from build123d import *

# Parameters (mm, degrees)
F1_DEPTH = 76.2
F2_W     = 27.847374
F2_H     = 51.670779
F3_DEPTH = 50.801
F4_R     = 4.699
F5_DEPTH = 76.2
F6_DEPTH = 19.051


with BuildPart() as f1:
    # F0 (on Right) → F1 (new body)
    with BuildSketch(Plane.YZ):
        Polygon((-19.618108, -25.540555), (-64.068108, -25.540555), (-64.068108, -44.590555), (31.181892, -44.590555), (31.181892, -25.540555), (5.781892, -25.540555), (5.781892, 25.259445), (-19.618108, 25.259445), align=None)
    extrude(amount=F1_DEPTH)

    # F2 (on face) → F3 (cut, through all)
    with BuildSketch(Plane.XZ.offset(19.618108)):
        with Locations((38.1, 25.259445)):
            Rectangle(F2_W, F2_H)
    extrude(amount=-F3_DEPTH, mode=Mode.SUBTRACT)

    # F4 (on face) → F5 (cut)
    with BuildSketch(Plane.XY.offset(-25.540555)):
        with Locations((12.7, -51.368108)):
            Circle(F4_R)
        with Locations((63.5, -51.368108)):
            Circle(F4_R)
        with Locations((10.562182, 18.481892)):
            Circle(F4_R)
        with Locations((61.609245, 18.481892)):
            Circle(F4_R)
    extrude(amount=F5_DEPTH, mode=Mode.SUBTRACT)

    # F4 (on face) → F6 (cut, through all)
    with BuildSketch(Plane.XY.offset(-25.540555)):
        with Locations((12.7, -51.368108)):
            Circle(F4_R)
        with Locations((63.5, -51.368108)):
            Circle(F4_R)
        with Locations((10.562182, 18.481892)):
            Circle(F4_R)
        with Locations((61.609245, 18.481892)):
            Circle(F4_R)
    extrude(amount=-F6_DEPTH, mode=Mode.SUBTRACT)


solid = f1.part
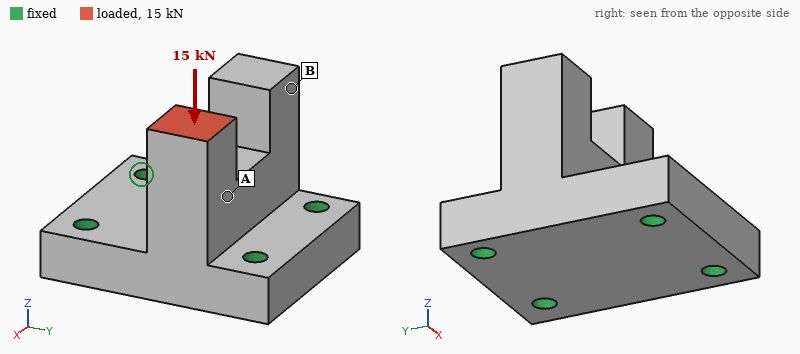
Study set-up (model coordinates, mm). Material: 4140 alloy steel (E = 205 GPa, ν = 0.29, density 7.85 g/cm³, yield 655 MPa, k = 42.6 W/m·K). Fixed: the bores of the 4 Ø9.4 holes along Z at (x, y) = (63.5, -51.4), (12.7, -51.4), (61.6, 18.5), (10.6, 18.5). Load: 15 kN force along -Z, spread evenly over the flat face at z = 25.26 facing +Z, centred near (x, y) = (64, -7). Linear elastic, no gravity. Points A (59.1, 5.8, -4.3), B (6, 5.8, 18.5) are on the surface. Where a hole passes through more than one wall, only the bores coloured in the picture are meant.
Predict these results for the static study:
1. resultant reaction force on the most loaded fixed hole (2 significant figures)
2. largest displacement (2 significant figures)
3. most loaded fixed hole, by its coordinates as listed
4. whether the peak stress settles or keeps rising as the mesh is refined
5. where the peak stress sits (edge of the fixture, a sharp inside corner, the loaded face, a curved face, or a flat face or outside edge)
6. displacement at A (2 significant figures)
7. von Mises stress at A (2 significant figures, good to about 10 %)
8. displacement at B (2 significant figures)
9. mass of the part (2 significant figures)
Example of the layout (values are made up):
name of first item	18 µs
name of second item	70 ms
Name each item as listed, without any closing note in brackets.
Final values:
resultant reaction force on the most loaded fixed hole	10 kN
largest displacement	20 µm
most loaded fixed hole, by its coordinates as listed	(61.6, 18.5)
whether the peak stress settles or keeps rising as the mesh is refined	keeps rising
where the peak stress sits	edge of the fixture
displacement at A	8.7 µm
von Mises stress at A	22 MPa
displacement at B	6.6 µm
mass of the part	1.7 kg
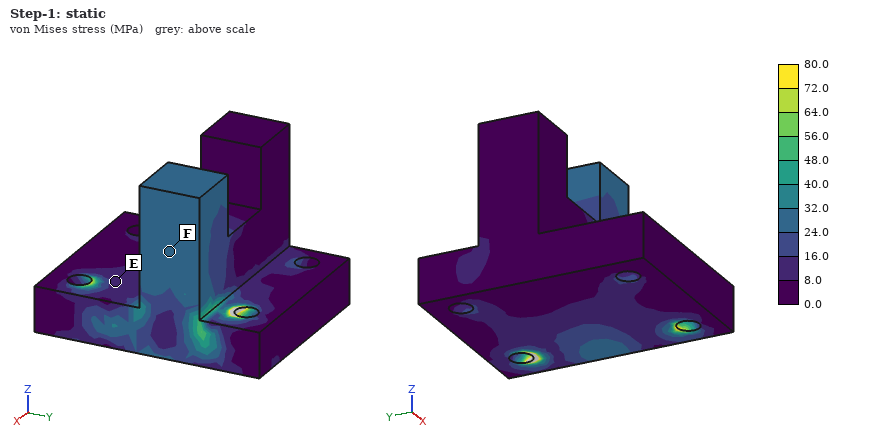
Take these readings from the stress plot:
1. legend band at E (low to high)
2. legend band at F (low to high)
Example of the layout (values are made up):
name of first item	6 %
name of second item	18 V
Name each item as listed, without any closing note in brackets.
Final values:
legend band at E	8.0 to 16.0 MPa
legend band at F	24.0 to 32.0 MPa
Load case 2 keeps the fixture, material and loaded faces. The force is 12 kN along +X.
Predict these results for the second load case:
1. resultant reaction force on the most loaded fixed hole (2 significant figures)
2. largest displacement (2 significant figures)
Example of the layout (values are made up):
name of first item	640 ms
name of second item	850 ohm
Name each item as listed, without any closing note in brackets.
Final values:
resultant reaction force on the most loaded fixed hole	10 kN
largest displacement	73 µm
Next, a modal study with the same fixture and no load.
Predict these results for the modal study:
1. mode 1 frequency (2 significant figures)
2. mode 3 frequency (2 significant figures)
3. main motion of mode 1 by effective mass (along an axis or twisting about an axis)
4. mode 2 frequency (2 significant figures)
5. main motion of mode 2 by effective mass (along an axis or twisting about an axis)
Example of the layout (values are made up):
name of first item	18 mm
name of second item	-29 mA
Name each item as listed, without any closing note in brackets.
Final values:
mode 1 frequency	5500 Hz
mode 3 frequency	7200 Hz
main motion of mode 1 by effective mass	along Y
mode 2 frequency	6200 Hz
main motion of mode 2 by effective mass	along X
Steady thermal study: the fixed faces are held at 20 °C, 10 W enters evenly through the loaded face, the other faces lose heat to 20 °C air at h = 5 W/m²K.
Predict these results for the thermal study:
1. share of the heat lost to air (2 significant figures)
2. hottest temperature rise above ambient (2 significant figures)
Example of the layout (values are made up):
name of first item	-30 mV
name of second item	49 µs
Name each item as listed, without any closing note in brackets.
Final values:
share of the heat lost to air	4.2 %
hottest temperature rise above ambient	20 K
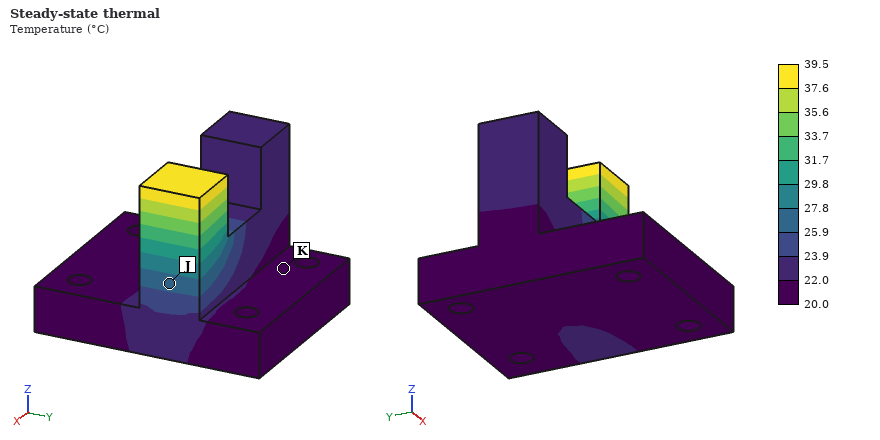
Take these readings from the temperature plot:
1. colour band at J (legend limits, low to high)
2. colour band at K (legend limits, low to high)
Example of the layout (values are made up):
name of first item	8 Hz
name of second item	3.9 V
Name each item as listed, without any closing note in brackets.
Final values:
colour band at J	25.9 to 27.8 °C
colour band at K	20.0 to 22.0 °C
